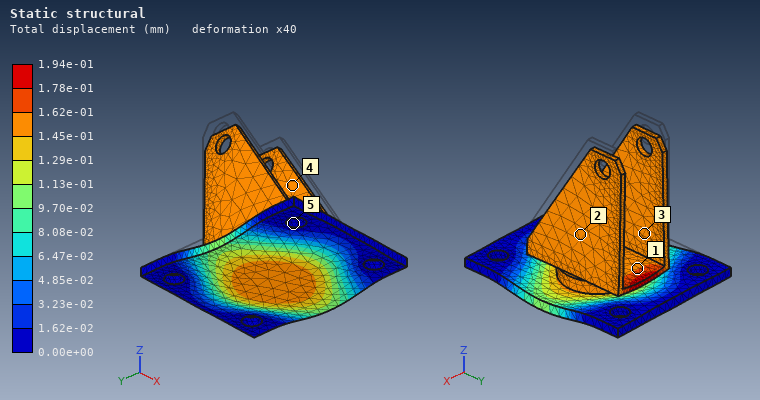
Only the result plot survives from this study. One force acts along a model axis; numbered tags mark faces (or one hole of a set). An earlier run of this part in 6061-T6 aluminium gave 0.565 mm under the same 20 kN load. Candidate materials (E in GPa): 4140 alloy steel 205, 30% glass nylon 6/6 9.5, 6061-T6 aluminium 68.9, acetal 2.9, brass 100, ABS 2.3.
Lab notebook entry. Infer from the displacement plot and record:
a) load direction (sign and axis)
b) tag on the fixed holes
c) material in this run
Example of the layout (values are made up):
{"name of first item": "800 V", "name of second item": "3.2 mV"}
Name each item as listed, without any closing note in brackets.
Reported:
{"load direction": "-Z", "tag on the fixed holes": "5", "material in this run": "4140 alloy steel"}
